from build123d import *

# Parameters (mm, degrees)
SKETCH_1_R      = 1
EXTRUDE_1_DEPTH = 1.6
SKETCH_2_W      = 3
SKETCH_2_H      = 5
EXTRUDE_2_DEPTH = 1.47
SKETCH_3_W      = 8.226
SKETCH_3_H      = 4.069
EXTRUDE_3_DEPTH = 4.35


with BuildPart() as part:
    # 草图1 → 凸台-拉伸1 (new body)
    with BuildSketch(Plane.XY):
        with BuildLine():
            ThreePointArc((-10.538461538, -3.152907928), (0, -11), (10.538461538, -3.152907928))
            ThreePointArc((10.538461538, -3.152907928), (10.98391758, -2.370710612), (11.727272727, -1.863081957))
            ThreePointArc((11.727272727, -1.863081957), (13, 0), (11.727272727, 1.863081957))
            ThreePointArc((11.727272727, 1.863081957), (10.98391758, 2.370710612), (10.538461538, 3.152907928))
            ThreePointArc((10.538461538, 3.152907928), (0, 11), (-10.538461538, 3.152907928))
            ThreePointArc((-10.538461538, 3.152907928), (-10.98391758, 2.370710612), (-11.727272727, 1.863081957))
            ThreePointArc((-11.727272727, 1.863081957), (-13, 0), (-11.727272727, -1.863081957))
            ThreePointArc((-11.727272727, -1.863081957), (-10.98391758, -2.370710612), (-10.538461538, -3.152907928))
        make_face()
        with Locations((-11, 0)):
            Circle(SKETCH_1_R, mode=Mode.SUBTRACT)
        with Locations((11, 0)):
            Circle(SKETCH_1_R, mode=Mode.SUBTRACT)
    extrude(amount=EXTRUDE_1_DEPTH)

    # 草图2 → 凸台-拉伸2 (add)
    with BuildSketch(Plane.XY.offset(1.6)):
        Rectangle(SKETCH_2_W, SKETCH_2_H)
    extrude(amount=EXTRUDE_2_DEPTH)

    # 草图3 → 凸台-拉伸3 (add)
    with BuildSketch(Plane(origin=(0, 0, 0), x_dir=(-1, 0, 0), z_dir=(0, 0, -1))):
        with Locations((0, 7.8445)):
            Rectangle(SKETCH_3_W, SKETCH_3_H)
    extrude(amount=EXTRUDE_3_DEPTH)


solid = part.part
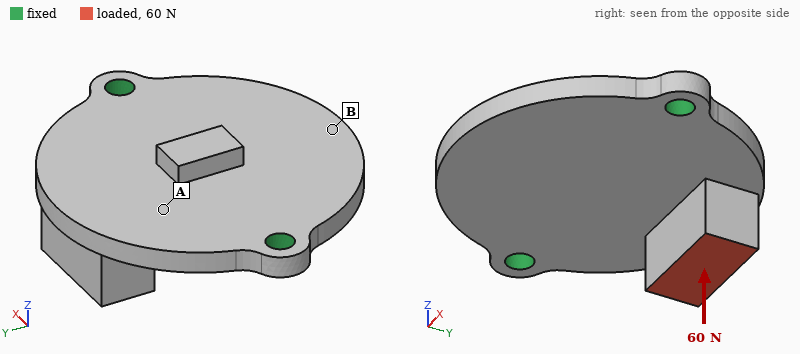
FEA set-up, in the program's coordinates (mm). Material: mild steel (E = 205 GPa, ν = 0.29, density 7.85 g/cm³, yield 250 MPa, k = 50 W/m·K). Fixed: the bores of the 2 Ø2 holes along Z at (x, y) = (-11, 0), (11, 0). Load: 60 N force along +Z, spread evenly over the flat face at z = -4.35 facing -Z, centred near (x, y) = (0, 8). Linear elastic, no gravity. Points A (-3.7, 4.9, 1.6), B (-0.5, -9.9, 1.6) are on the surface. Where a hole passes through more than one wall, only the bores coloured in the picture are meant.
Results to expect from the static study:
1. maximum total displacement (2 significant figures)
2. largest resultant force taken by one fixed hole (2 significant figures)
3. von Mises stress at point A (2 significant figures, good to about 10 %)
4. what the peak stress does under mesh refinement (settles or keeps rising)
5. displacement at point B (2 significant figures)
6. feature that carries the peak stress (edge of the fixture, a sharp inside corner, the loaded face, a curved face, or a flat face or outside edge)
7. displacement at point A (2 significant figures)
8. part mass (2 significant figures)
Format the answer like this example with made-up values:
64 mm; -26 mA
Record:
22 µm; 30 N; 30 MPa; keeps rising; 7.8 µm; edge of the fixture; 9.2 µm; 6.2 g
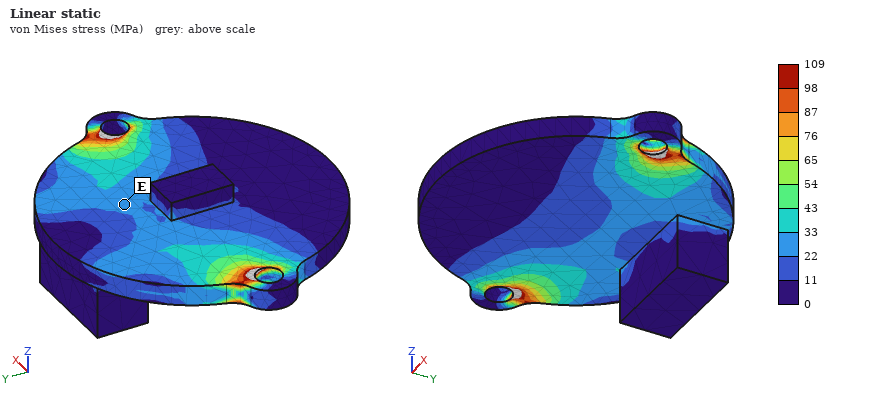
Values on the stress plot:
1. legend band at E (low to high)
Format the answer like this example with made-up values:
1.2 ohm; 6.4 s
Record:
22 to 33 MPa
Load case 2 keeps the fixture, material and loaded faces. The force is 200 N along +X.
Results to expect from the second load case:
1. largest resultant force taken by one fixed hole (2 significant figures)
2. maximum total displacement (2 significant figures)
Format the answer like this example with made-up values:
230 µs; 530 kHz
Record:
140 N; 12 µm
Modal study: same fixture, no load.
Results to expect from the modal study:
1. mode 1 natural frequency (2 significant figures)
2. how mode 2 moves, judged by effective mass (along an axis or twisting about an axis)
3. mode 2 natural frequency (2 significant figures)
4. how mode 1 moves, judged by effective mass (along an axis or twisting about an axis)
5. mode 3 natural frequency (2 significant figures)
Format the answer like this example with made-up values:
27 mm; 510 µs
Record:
6100 Hz; along Z; 9900 Hz; along Z; 21 kHz
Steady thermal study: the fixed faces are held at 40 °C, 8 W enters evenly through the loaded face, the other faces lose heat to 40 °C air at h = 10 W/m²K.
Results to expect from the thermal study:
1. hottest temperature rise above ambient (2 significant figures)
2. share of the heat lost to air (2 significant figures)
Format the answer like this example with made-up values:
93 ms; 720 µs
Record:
87 K; 4.4 %
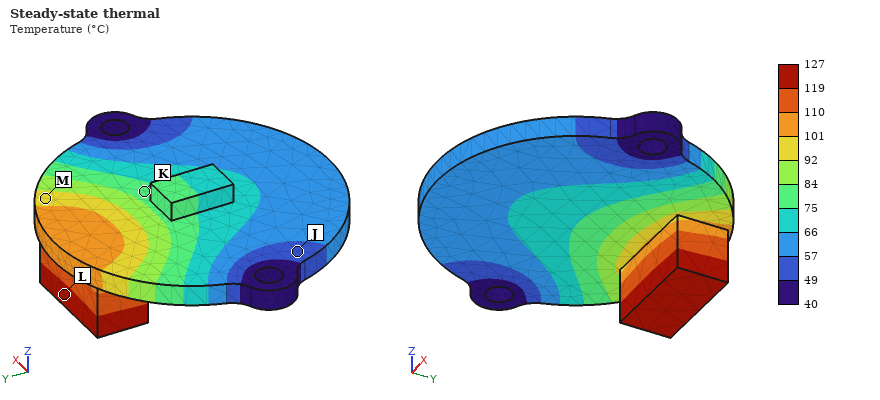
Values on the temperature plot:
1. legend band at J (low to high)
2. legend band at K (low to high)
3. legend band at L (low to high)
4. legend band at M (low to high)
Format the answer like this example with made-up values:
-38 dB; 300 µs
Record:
49 to 57 °C; 75 to 84 °C; 119 to 127 °C; 92 to 101 °C
